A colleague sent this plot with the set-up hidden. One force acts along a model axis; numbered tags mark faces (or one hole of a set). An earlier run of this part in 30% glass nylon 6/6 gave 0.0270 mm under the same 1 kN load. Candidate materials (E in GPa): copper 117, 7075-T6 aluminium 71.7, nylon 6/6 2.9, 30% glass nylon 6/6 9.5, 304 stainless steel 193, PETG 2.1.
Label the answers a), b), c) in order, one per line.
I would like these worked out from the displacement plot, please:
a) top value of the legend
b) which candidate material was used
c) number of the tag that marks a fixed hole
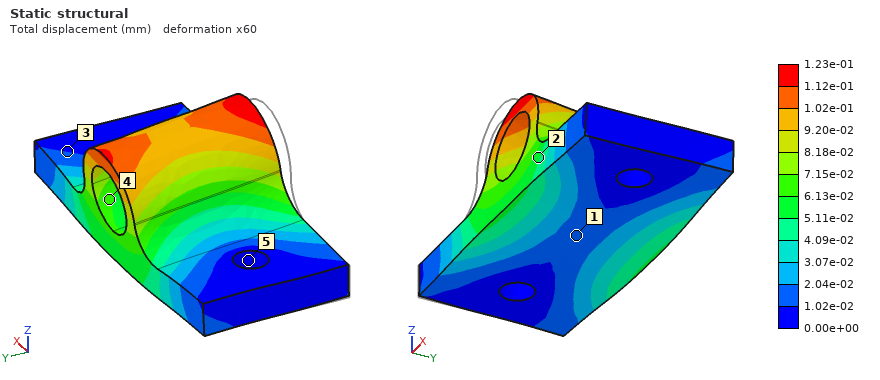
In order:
a) 1.23e-01 mm
b) PETG
c) 5
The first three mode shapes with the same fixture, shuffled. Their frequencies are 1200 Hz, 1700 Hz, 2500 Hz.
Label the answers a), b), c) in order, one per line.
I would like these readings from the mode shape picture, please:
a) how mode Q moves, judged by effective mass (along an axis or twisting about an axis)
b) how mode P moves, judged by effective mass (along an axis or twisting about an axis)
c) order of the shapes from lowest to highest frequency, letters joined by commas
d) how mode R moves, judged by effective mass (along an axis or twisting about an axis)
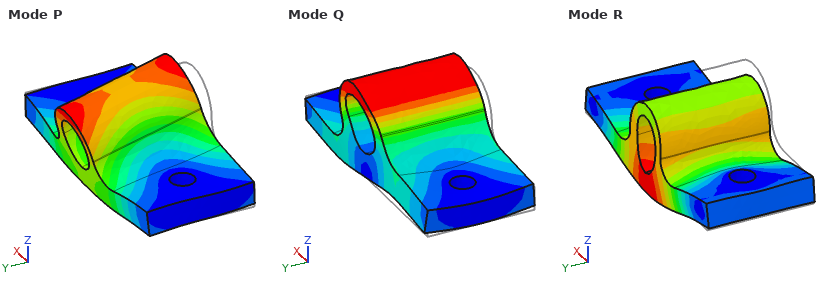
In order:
a) along X
b) along Y
c) P, R, Q
d) along Z
